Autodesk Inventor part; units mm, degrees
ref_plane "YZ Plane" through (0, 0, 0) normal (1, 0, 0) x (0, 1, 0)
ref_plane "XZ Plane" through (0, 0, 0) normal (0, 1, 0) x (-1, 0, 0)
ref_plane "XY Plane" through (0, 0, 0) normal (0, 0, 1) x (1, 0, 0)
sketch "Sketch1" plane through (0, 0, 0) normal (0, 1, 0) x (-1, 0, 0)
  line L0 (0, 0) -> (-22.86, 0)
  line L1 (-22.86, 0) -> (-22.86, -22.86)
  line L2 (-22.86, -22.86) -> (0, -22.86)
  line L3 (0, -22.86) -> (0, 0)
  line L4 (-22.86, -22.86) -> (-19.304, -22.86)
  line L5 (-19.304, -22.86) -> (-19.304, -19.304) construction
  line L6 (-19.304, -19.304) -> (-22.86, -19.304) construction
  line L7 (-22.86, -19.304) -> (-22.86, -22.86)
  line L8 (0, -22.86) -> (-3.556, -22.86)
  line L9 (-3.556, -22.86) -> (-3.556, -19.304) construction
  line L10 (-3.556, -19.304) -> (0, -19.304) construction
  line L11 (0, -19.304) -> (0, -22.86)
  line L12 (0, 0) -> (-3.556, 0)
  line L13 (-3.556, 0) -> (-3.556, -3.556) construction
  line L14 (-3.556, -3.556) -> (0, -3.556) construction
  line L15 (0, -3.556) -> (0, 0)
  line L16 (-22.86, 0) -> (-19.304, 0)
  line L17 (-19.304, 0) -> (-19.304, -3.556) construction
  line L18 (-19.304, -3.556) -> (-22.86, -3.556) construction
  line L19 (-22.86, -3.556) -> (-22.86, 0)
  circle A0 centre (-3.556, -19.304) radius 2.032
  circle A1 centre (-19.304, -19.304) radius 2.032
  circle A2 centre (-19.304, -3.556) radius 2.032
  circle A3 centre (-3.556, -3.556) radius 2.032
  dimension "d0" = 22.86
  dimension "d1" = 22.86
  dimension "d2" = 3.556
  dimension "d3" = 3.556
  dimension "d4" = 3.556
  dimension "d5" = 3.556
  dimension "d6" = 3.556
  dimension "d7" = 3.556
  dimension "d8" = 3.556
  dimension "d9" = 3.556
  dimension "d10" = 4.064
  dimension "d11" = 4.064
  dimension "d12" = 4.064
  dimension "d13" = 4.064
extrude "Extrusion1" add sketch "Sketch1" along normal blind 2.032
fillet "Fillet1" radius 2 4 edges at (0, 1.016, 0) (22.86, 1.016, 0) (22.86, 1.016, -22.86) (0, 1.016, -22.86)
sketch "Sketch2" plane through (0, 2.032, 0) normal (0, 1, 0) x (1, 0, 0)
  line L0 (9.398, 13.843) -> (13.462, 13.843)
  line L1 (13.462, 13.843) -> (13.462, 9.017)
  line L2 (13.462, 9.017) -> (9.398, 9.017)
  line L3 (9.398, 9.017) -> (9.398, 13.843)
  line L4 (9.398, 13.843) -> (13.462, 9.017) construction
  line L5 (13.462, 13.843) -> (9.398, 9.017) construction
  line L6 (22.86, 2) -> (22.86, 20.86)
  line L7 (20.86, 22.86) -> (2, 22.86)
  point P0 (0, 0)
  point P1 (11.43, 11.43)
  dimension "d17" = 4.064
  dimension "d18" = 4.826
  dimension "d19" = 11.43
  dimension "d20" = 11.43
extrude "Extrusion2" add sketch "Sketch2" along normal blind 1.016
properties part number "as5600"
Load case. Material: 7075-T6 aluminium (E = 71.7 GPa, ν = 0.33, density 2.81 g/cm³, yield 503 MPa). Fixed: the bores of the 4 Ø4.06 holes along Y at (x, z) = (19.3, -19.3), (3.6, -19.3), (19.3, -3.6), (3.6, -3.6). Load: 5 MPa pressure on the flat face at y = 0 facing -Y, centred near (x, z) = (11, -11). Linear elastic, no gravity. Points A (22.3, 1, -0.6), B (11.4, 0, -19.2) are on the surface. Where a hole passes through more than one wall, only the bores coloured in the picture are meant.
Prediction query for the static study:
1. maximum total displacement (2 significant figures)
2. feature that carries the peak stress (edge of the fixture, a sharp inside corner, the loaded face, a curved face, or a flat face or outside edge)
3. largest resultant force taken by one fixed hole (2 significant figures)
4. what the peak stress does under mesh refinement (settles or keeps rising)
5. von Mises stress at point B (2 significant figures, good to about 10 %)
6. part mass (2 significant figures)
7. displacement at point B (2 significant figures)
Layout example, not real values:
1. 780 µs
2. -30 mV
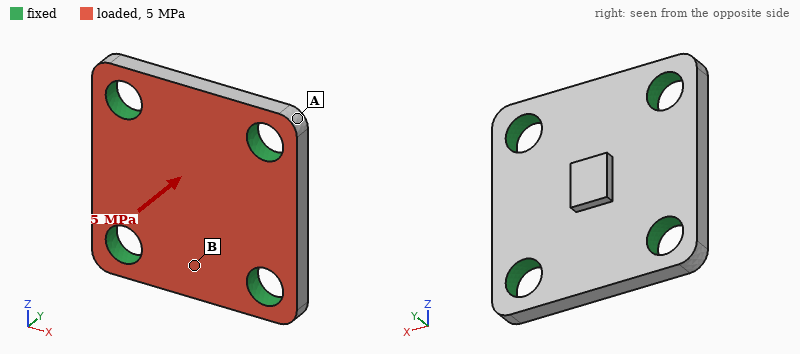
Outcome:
1. 19 µm
2. edge of the fixture
3. 580 N
4. keeps rising
5. 55 MPa
6. 2.7 g
7. 11 µm
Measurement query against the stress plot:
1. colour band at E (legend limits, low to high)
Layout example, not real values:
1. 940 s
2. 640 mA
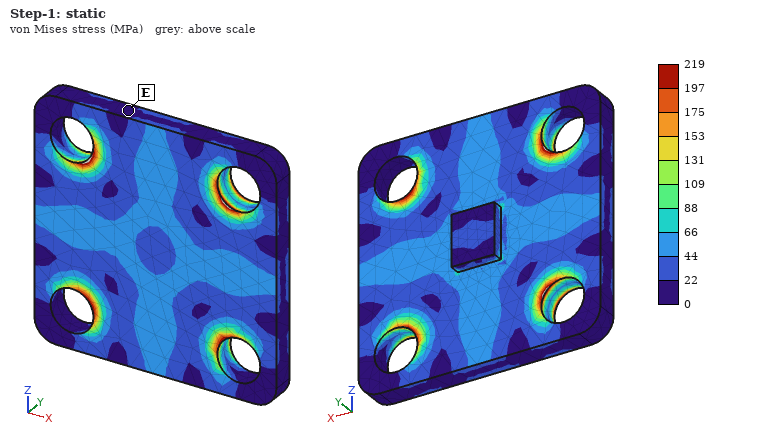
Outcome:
1. 0 to 22 MPa
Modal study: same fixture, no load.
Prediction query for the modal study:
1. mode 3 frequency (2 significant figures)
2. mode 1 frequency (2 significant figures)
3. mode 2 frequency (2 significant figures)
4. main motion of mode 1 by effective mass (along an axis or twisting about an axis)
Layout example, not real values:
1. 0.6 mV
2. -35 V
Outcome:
1. 58 kHz
2. 39 kHz
3. 58 kHz
4. along Y
